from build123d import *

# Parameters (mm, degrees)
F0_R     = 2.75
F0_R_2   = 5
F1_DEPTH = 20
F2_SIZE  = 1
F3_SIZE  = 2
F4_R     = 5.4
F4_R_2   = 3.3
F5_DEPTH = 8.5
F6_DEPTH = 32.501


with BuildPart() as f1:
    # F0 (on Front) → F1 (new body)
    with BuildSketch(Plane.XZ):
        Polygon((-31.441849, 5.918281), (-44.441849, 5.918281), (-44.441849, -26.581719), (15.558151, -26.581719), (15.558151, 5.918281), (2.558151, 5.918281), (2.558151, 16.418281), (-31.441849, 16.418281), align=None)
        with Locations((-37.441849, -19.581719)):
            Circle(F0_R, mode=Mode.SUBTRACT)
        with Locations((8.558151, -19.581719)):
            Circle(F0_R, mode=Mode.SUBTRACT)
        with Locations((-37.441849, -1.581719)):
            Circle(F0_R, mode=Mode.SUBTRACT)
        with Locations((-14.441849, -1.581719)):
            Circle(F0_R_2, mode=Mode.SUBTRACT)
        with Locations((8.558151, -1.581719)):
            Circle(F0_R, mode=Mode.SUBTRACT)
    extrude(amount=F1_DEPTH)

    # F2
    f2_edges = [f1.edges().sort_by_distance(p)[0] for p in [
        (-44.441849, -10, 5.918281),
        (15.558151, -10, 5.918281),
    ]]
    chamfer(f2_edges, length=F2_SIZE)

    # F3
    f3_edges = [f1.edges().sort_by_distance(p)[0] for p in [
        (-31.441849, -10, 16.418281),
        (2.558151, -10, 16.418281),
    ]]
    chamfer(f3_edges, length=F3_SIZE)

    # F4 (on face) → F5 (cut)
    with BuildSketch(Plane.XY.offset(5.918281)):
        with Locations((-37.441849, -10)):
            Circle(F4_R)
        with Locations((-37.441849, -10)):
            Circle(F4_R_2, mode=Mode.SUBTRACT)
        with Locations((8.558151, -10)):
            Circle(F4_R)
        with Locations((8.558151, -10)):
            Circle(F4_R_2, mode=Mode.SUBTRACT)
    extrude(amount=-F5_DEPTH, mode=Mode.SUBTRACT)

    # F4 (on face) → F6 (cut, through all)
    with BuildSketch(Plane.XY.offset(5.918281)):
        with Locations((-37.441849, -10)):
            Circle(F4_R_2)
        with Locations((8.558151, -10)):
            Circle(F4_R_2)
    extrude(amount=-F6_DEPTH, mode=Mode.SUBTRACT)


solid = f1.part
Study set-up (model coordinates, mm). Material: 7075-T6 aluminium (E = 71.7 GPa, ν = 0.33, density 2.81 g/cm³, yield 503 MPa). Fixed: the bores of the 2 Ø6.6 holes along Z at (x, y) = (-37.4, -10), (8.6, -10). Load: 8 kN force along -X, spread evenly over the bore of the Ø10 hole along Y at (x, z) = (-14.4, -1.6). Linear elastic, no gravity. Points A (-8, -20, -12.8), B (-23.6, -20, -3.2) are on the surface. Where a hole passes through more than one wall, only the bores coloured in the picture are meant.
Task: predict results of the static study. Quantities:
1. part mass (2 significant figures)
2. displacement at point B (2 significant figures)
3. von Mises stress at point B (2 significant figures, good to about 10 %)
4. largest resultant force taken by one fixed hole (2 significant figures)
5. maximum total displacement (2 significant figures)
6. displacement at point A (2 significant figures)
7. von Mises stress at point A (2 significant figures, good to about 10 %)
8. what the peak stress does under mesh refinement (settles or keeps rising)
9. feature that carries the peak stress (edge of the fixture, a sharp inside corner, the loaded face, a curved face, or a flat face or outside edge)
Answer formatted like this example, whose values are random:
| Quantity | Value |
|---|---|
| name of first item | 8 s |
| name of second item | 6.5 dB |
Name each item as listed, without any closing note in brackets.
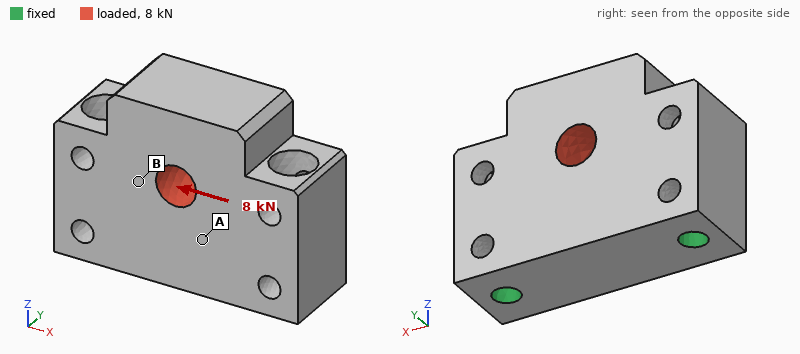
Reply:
| Quantity | Value |
|---|---|
| part mass | 110 g |
| displacement at point B | 3.4 µm |
| von Mises stress at point B | 16 MPa |
| largest resultant force taken by one fixed hole | 4.3 kN |
| maximum total displacement | 6.3 µm |
| displacement at point A | 1.5 µm |
| von Mises stress at point A | 6.2 MPa |
| what the peak stress does under mesh refinement | keeps rising |
| feature that carries the peak stress | edge of the fixture |
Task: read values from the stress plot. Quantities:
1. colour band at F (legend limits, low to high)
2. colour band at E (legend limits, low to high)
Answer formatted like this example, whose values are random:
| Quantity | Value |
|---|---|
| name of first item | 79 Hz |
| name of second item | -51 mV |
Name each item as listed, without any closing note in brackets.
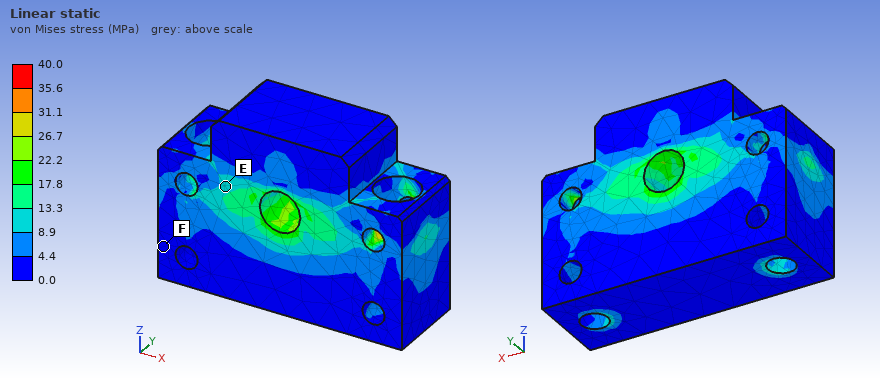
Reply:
| Quantity | Value |
|---|---|
| colour band at F | 0.0 to 4.4 MPa |
| colour band at E | 8.9 to 13.3 MPa |
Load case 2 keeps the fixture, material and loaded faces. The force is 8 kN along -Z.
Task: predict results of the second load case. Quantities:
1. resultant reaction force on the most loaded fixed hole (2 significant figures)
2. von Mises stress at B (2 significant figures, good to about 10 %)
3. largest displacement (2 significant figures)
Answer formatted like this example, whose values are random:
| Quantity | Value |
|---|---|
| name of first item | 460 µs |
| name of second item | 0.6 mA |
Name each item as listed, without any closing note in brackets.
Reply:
| Quantity | Value |
|---|---|
| resultant reaction force on the most loaded fixed hole | 4.2 kN |
| von Mises stress at B | 8.8 MPa |
| largest displacement | 7.0 µm |
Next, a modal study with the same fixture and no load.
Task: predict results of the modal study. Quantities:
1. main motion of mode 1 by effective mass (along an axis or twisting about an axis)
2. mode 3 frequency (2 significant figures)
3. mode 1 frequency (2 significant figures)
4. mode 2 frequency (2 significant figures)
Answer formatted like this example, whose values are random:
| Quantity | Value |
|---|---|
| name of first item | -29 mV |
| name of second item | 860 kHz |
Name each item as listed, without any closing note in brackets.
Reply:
| Quantity | Value |
|---|---|
| main motion of mode 1 by effective mass | along Y |
| mode 3 frequency | 24 kHz |
| mode 1 frequency | 12 kHz |
| mode 2 frequency | 24 kHz |
